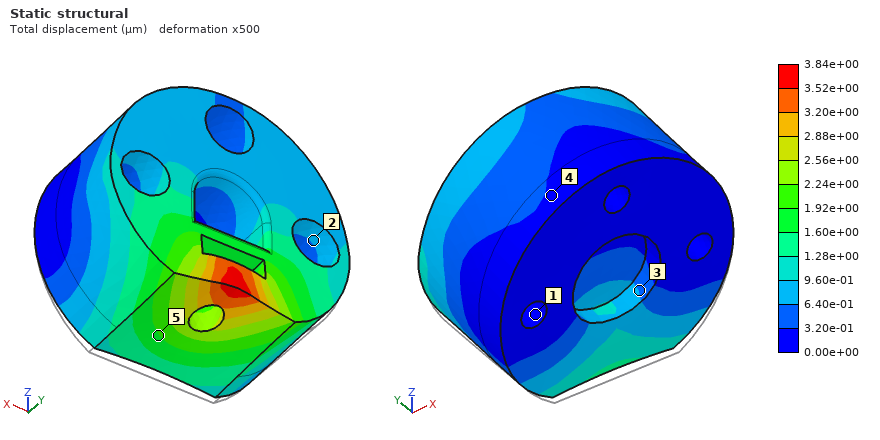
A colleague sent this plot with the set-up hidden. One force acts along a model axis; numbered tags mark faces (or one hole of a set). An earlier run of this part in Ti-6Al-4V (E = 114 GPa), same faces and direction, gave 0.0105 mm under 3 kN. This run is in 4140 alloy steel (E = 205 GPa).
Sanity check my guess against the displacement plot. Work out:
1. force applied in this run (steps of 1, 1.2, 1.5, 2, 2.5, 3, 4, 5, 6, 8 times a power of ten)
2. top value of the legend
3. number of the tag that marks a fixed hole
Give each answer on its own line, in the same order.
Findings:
2 kN
3.84e+00 µm
1
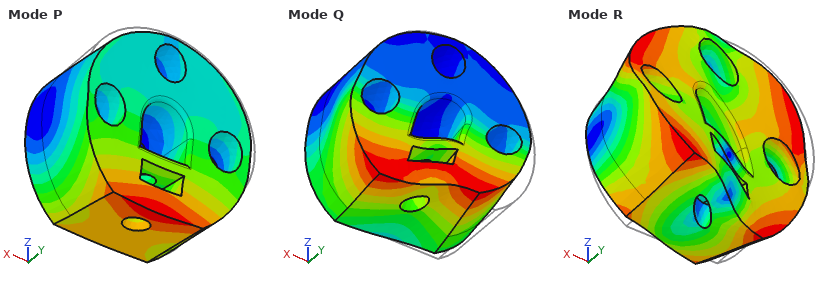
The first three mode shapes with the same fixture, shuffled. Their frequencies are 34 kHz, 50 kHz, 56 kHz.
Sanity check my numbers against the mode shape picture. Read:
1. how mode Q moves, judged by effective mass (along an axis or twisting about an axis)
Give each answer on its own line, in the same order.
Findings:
along X
